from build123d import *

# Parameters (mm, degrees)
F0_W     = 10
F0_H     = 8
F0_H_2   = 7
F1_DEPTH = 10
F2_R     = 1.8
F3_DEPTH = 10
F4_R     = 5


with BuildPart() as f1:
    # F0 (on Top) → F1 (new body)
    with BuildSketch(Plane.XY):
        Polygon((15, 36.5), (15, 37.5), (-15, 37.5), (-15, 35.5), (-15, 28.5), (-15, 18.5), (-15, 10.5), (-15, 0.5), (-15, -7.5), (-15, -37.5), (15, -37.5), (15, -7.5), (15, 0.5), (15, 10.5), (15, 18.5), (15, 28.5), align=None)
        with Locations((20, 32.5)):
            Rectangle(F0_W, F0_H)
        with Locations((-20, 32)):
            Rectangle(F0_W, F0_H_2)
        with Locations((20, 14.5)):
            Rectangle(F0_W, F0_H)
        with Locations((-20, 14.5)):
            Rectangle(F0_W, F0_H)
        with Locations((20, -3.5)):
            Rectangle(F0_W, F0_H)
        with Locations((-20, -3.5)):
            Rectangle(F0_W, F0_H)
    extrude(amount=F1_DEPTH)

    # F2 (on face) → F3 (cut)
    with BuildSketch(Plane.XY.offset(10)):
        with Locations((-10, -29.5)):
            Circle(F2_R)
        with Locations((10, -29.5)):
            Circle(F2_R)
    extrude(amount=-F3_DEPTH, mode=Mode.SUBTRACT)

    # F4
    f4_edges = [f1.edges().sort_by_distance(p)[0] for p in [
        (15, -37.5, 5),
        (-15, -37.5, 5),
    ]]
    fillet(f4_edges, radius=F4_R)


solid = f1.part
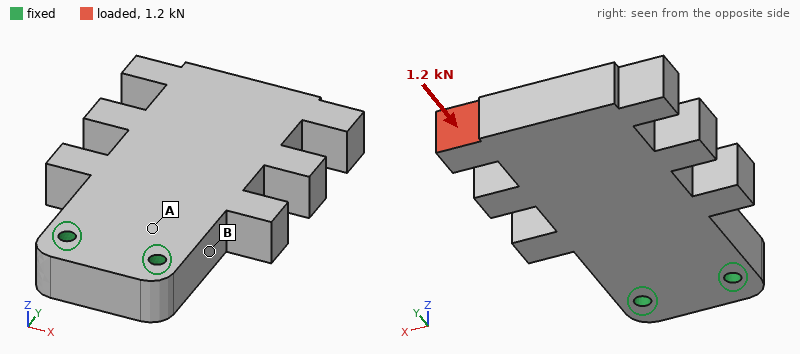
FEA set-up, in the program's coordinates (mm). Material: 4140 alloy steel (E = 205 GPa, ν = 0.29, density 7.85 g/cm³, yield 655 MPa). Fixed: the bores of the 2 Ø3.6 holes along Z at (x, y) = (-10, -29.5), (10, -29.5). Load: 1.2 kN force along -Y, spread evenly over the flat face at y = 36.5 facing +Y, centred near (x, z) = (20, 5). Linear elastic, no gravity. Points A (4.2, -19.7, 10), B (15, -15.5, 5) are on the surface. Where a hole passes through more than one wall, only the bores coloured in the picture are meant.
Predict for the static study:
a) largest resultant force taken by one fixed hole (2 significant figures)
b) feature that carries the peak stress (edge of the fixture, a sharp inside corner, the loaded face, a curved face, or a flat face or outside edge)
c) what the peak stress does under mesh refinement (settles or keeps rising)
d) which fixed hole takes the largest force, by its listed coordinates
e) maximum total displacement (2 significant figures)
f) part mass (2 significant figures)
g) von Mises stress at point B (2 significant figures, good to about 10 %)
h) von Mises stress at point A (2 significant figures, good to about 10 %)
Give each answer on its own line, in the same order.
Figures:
1.7 kN
a sharp inside corner
keeps rising
(10, -29.5)
21 µm
210 g
20 MPa
7.9 MPa
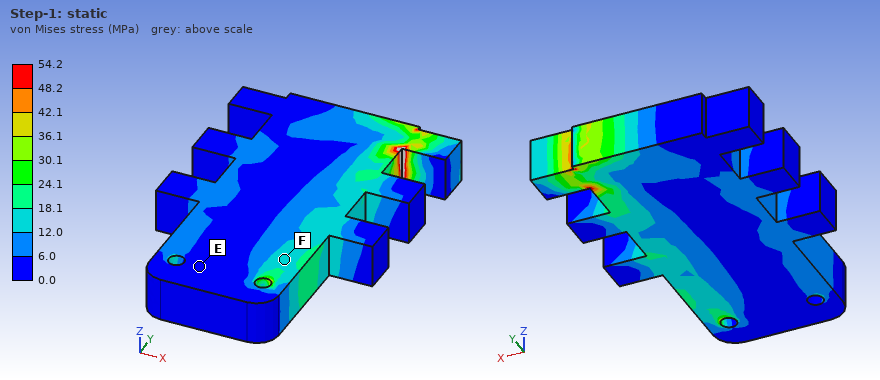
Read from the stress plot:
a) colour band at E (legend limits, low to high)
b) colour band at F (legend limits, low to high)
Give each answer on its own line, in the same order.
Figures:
0.0 to 6.0 MPa
12.0 to 18.1 MPa
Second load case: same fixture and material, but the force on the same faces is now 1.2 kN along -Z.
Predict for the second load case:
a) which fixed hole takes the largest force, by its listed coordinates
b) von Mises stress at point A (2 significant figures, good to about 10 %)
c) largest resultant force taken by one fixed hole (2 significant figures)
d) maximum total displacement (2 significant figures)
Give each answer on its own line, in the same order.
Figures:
(10, -29.5)
130 MPa
1.6 kN
0.30 mm
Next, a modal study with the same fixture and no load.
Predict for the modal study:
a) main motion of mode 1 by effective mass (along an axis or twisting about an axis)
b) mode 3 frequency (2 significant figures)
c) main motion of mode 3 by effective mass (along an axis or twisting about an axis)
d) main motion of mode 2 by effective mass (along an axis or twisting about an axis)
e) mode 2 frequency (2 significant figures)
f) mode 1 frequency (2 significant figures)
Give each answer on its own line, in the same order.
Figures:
along Z
4600 Hz
twisting about Y
along X
4000 Hz
1500 Hz
